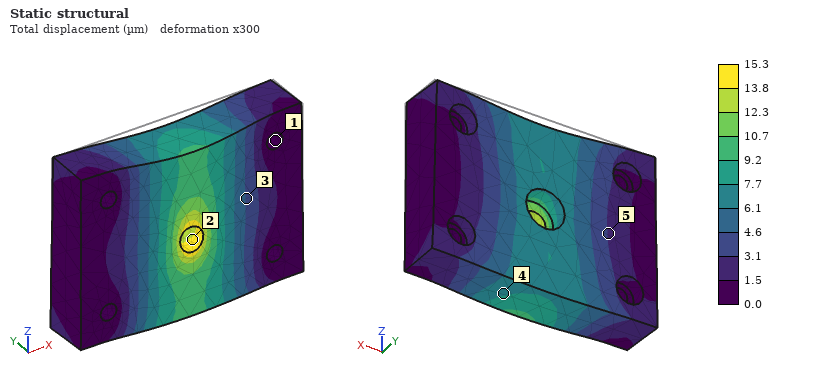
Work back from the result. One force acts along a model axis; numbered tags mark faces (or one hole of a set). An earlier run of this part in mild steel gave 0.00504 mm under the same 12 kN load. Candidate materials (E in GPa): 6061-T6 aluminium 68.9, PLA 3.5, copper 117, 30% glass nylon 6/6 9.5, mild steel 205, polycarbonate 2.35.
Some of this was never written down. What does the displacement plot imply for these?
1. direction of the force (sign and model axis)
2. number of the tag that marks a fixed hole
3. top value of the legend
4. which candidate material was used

-Z
1
15.3 µm
6061-T6 aluminium
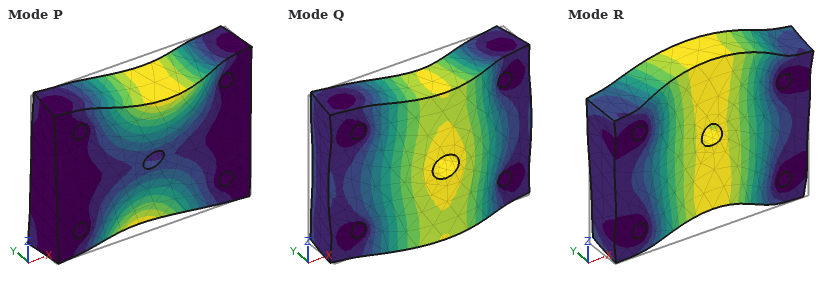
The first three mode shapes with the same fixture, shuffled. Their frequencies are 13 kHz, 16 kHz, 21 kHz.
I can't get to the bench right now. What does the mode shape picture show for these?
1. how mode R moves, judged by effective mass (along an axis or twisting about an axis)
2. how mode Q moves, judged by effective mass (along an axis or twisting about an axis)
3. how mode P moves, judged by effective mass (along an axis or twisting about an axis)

along Z
along Y
twisting about X
